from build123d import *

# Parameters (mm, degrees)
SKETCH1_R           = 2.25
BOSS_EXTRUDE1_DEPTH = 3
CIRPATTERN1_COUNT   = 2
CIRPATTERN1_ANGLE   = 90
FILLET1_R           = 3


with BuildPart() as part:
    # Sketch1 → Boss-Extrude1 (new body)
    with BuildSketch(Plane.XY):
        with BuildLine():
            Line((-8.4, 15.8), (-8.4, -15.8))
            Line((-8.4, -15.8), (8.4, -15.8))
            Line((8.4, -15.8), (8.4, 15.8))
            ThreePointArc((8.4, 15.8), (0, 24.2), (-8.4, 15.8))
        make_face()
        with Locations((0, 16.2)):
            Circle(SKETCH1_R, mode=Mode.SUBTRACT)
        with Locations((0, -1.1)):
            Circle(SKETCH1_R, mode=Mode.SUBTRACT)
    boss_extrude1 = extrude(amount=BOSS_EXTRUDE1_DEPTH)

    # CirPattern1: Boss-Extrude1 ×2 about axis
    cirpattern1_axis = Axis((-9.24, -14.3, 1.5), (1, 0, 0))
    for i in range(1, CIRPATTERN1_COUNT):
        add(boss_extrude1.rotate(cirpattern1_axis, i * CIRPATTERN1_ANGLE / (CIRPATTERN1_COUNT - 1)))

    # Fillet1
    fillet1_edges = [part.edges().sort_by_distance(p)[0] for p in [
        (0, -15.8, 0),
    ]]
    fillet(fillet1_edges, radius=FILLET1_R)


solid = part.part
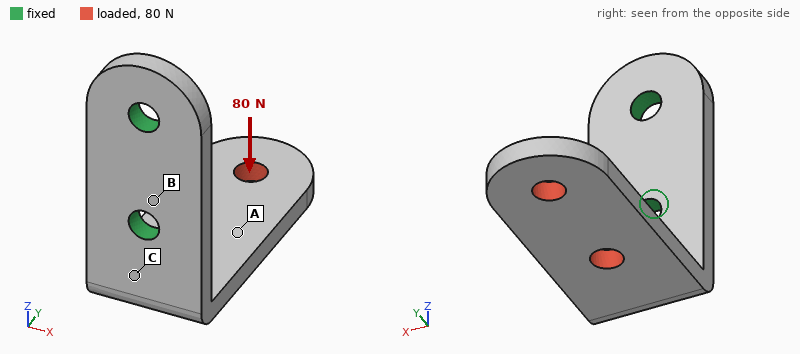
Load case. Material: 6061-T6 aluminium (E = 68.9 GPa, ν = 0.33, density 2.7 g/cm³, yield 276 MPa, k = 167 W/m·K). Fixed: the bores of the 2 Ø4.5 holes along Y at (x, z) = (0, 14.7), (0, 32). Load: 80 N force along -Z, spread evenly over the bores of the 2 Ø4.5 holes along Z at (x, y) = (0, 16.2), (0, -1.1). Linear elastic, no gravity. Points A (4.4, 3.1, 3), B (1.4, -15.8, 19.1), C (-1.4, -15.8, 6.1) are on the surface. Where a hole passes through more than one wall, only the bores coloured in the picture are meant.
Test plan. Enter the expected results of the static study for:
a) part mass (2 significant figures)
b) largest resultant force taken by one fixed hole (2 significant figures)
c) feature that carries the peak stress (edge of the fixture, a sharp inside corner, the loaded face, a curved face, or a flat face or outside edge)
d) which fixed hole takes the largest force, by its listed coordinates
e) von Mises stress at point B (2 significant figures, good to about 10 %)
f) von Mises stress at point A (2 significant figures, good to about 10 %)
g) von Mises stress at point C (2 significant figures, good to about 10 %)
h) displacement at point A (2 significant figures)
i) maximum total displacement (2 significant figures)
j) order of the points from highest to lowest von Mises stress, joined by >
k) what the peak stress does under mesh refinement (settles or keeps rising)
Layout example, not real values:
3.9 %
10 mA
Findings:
9.4 g
73 N
edge of the fixture
(0, 14.7)
8.7 MPa
23 MPa
60 MPa
0.21 mm
0.55 mm
C > A > B
keeps rising
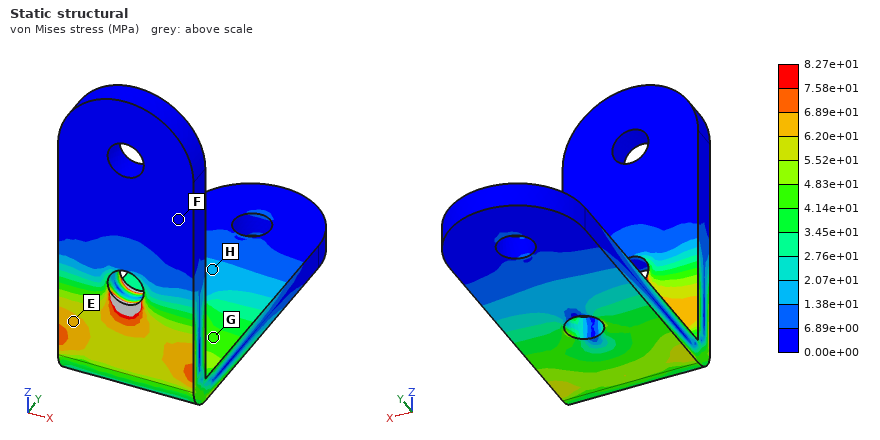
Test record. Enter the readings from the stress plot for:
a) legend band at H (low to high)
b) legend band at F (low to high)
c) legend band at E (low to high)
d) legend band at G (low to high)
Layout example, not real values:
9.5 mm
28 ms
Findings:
1.38e+01 to 2.07e+01 MPa
0.00e+00 to 6.89e+00 MPa
6.20e+01 to 6.89e+01 MPa
4.14e+01 to 4.83e+01 MPa
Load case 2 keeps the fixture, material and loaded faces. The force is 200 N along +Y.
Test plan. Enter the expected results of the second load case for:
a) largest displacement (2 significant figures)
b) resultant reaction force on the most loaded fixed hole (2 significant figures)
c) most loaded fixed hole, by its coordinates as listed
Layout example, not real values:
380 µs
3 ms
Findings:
0.23 mm
220 N
(0, 14.7)
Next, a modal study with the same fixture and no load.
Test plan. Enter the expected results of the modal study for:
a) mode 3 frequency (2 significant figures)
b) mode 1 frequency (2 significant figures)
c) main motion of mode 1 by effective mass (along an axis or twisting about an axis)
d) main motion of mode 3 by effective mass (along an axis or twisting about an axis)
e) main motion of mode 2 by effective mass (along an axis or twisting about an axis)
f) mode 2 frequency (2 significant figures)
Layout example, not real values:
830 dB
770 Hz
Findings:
5500 Hz
1200 Hz
along Z
along Y
along X
2000 Hz
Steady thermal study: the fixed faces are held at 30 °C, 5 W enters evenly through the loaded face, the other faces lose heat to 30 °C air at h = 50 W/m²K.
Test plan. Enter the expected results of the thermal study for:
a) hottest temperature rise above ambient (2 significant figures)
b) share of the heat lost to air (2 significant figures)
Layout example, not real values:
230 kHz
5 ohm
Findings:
18 K
20 %
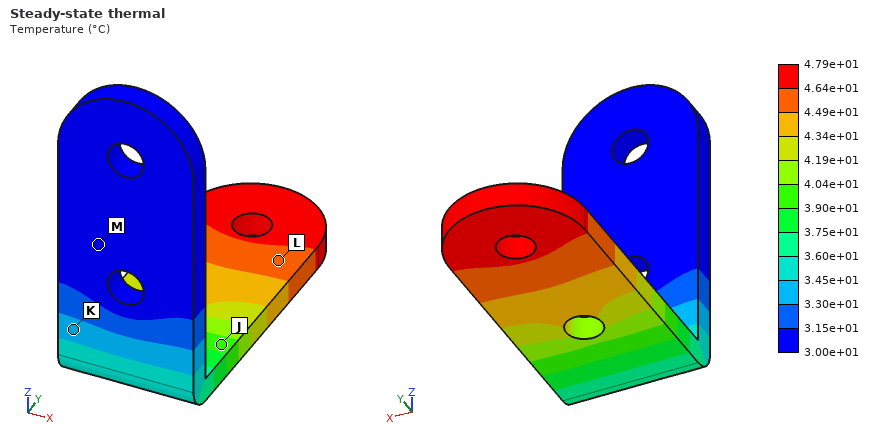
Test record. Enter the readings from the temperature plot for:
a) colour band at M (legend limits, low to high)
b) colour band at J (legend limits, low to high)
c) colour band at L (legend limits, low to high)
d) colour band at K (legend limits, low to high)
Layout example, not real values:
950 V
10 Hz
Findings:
3.00e+01 to 3.15e+01 °C
3.90e+01 to 4.04e+01 °C
4.49e+01 to 4.64e+01 °C
3.30e+01 to 3.45e+01 °C
